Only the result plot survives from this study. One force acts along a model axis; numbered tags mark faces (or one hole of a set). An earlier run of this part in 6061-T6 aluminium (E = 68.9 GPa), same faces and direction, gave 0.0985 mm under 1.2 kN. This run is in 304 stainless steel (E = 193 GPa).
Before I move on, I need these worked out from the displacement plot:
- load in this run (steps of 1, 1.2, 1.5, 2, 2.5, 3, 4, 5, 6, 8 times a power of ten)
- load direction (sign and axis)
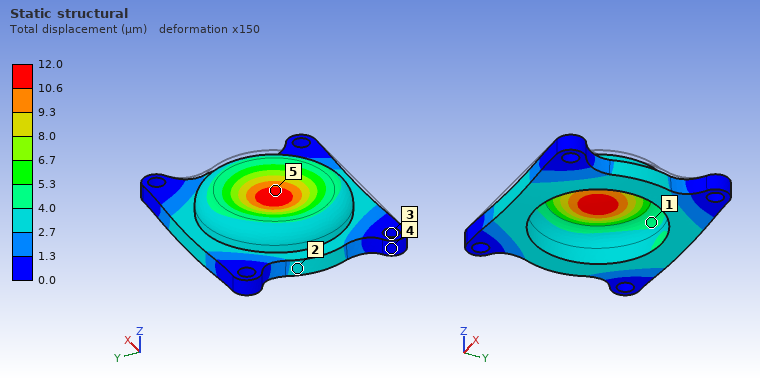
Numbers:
400 N
-Z
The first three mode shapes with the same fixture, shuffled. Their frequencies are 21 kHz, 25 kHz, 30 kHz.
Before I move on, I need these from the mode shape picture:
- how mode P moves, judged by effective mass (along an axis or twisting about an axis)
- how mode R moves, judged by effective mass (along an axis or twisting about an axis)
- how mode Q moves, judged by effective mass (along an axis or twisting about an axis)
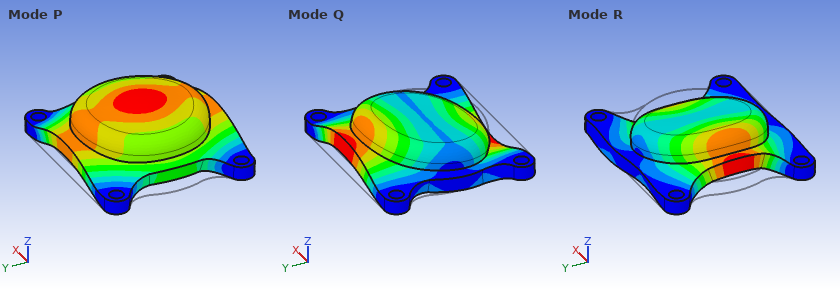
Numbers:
along Z
twisting about Y
twisting about X
